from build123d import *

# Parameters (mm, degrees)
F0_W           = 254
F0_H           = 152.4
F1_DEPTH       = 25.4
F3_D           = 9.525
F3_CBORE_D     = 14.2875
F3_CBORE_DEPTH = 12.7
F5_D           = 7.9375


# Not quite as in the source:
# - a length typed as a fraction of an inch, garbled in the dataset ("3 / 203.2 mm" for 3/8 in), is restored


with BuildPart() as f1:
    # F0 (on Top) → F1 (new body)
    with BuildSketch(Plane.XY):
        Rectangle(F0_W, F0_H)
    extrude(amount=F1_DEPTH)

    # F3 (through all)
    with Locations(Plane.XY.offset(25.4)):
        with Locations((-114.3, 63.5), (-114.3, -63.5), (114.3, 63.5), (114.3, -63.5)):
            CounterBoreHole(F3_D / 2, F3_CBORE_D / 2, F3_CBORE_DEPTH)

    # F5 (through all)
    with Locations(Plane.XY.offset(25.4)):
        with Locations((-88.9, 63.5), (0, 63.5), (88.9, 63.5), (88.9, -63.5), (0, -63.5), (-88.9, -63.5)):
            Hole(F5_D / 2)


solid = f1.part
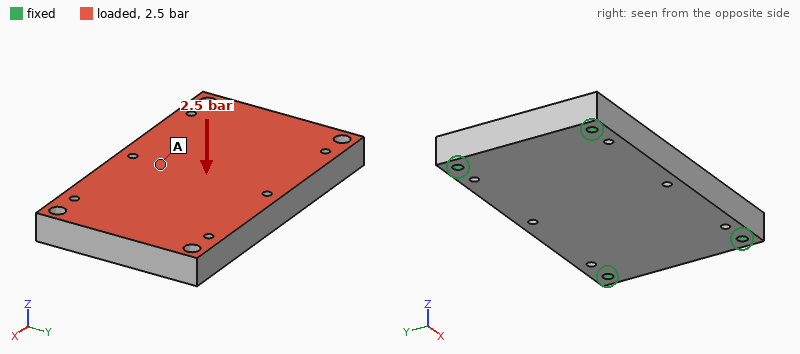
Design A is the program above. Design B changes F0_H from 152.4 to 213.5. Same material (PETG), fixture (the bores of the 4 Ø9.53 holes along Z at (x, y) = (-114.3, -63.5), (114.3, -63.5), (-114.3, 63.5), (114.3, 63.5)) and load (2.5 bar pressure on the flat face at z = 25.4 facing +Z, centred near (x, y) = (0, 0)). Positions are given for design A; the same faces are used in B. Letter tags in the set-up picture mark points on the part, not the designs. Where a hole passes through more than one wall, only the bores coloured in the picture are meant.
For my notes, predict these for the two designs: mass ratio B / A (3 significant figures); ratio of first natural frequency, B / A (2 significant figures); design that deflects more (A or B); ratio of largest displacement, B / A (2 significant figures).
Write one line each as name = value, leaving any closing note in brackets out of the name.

mass ratio B / A = 1.41
ratio of first natural frequency, B / A = 0.96
design that deflects more = B
ratio of largest displacement, B / A = 1.1
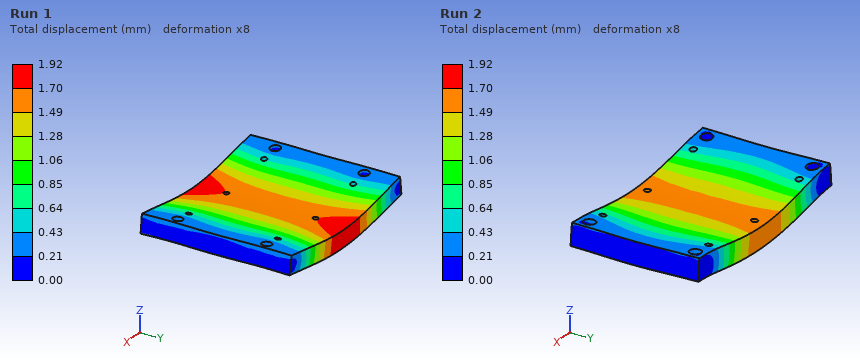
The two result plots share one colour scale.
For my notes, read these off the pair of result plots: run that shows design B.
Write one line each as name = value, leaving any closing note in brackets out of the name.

run that shows design B = Run 1
